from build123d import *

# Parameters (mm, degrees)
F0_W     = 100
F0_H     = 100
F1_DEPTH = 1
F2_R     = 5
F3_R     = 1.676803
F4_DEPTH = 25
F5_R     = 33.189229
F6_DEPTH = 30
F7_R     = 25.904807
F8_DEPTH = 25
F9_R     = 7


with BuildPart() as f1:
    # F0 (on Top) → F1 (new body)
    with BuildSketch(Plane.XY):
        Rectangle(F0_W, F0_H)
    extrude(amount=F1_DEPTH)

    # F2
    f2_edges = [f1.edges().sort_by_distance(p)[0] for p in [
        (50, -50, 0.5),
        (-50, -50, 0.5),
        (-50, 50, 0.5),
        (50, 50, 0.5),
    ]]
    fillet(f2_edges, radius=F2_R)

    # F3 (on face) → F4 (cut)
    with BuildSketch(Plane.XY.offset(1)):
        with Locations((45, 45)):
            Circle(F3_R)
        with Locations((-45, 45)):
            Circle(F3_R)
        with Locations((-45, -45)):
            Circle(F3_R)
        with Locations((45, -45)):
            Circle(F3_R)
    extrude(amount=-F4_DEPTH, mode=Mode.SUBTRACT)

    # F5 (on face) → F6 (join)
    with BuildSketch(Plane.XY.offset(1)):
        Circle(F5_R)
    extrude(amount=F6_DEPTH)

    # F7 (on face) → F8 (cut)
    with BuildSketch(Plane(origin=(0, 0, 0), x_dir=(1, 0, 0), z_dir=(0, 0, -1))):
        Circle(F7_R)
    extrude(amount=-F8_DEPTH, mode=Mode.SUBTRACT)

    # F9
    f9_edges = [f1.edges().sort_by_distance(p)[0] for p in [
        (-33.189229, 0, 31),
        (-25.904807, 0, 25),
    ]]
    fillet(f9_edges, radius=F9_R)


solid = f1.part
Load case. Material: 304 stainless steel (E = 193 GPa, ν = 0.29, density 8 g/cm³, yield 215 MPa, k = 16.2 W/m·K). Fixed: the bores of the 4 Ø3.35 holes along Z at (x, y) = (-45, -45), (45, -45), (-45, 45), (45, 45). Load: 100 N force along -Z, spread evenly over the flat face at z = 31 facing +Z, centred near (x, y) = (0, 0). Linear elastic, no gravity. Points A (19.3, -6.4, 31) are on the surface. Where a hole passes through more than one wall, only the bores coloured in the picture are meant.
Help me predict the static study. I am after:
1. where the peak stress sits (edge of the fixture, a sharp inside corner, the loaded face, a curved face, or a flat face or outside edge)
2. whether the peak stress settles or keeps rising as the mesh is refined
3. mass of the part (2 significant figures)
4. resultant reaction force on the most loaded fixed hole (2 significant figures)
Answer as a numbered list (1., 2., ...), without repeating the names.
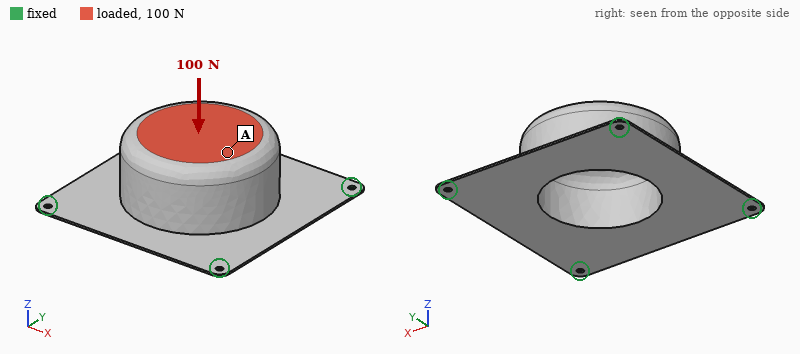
1. edge of the fixture
2. keeps rising
3. 480 g
4. 30 N
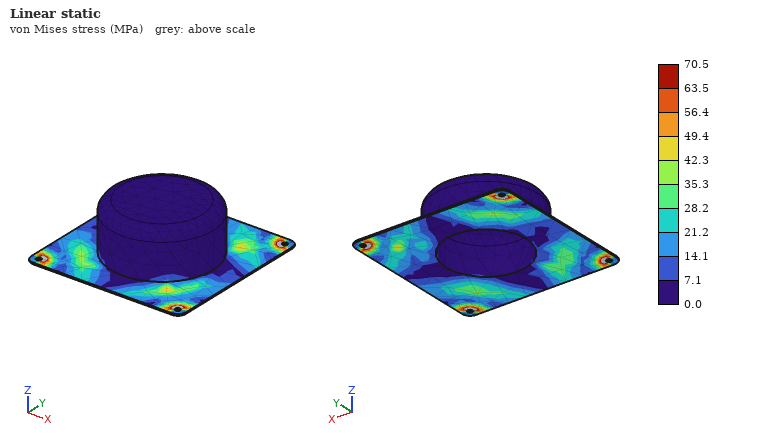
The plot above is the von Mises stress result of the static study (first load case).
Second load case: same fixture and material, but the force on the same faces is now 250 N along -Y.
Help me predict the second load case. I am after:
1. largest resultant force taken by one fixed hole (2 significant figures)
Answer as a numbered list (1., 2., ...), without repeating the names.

1. 90 N
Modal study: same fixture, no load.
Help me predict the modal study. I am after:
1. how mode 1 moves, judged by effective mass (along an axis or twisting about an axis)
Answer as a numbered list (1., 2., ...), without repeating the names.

1. along Z
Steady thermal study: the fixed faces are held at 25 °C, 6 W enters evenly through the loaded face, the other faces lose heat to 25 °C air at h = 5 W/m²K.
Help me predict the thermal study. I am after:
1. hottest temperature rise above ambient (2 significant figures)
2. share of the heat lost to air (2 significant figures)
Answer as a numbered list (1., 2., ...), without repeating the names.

1. 46 K
2. 72 %
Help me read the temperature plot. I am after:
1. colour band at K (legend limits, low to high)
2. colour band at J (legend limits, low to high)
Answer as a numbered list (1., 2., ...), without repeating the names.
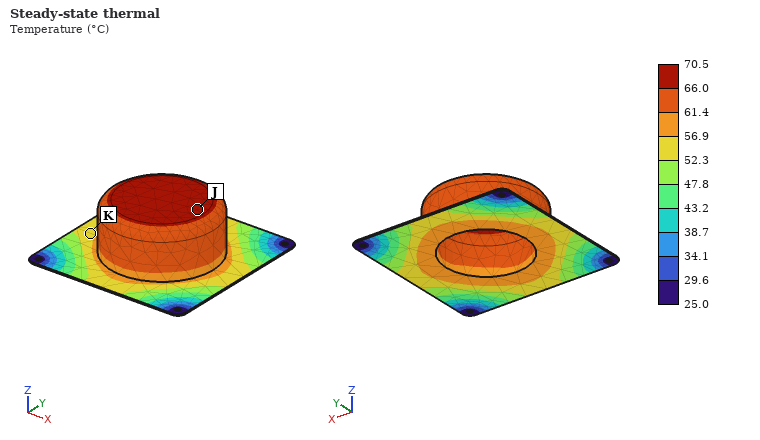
1. 52.3 to 56.9 °C
2. 66.0 to 70.5 °C
